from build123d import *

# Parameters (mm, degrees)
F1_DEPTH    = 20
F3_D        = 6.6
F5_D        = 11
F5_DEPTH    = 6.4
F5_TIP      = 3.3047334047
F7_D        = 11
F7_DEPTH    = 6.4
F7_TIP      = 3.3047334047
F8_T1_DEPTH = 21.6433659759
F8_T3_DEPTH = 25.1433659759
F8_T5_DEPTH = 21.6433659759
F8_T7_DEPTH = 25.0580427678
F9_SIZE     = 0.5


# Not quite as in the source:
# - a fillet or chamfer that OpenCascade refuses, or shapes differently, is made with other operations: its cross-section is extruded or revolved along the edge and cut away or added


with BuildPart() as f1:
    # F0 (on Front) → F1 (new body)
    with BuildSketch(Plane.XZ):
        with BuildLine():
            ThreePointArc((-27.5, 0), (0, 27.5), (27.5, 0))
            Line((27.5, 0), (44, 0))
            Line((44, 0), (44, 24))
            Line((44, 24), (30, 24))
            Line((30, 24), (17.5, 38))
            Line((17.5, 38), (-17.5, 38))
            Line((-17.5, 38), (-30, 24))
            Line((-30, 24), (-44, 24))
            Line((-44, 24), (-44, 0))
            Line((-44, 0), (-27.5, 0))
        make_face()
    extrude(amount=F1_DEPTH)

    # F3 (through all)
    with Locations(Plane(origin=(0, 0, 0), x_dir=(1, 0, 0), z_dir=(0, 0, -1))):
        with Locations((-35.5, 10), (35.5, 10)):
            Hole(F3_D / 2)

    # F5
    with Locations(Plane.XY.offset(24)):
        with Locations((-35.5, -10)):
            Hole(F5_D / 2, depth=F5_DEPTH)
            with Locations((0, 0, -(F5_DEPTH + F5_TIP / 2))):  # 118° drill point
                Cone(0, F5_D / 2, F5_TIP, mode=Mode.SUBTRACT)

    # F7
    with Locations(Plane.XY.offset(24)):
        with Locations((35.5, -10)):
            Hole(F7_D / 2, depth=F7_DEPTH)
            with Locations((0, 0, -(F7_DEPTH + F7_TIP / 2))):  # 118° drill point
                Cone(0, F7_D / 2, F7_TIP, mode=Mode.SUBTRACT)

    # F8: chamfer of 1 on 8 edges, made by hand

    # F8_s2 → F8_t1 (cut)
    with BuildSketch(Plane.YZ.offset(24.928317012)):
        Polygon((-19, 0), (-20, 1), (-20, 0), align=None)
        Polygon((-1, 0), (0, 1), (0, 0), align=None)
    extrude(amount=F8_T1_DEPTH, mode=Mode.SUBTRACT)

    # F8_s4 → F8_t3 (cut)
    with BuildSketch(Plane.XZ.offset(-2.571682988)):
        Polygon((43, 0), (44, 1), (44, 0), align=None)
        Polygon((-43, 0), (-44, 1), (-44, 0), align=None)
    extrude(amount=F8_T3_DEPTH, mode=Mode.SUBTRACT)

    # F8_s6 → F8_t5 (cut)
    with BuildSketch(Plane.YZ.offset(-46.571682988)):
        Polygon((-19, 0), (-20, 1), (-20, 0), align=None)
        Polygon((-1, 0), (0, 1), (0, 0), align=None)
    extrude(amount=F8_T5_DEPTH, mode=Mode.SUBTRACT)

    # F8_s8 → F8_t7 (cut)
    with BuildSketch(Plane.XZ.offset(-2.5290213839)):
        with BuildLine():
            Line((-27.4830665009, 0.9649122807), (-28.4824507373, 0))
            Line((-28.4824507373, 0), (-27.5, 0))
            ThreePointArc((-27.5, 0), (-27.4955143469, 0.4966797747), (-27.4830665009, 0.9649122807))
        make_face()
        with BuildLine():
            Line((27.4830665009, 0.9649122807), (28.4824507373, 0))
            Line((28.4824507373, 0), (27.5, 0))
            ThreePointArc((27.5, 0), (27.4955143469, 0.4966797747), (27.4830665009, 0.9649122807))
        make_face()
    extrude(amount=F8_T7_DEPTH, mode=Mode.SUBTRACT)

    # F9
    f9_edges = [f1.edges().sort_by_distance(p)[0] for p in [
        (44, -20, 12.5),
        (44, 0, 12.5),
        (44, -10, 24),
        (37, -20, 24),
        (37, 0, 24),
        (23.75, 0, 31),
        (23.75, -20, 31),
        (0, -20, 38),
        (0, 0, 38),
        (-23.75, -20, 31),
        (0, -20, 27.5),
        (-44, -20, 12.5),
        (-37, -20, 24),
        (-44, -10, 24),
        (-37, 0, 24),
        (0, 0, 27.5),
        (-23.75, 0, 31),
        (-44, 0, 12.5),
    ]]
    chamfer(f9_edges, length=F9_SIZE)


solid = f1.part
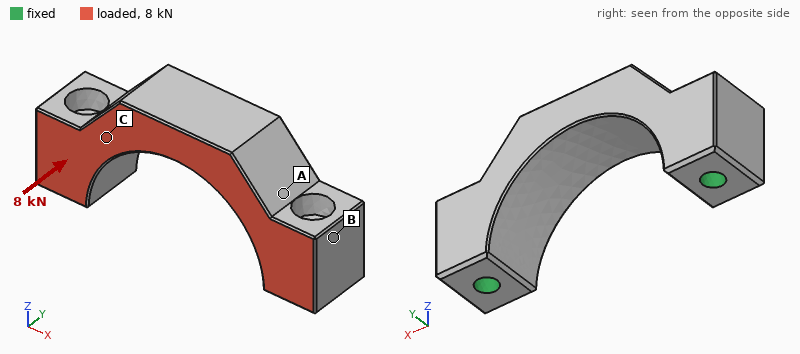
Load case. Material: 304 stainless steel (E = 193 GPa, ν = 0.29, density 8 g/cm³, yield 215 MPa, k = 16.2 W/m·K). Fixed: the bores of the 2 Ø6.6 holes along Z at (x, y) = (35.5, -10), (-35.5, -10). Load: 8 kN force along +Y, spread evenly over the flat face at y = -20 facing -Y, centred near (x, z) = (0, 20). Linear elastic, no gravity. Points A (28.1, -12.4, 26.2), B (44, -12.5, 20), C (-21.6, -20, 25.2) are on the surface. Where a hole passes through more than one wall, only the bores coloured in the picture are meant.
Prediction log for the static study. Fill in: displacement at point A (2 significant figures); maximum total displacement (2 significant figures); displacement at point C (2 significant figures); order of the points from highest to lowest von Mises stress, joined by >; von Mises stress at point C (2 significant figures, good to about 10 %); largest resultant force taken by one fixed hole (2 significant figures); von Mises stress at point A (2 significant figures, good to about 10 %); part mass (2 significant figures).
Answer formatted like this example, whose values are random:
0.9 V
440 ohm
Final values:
8.0 µm
20 µm
11 µm
A > C > B
17 MPa
4.0 kN
37 MPa
230 g
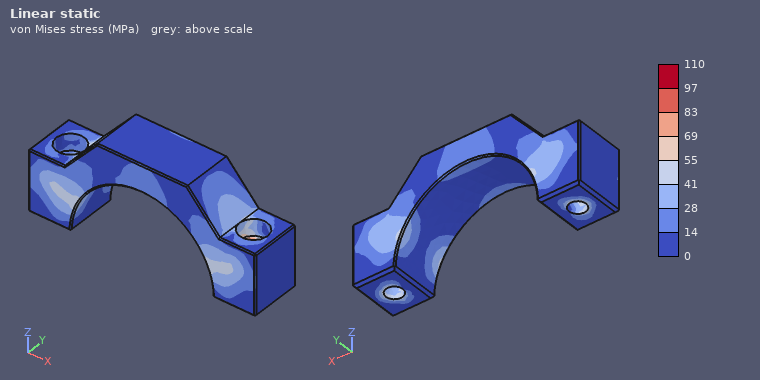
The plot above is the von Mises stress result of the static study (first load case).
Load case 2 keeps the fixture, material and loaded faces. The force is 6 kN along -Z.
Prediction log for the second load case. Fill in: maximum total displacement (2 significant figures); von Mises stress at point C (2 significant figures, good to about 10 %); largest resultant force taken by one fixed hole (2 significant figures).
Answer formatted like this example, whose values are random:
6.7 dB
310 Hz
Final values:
12 µm
25 MPa
3.2 kN
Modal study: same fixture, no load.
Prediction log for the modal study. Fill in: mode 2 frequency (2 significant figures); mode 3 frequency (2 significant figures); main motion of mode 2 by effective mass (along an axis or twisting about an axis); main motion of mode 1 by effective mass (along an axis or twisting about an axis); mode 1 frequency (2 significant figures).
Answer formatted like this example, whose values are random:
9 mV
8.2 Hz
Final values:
15 kHz
17 kHz
along X
along Y
7700 Hz
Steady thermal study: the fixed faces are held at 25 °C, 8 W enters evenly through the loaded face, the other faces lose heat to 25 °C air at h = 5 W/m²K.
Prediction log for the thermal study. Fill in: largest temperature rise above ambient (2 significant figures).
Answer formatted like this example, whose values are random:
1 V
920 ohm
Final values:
16 K
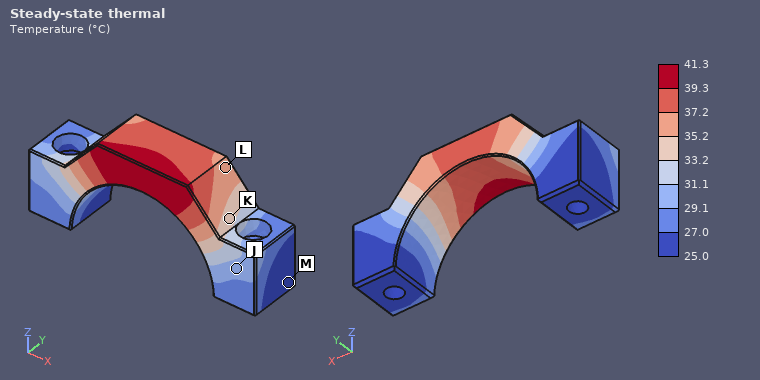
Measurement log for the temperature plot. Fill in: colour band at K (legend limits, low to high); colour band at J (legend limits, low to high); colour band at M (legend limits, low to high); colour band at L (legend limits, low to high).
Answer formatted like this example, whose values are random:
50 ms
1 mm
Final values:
33.2 to 35.2 °C
29.1 to 31.1 °C
25.0 to 27.0 °C
35.2 to 37.2 °C
